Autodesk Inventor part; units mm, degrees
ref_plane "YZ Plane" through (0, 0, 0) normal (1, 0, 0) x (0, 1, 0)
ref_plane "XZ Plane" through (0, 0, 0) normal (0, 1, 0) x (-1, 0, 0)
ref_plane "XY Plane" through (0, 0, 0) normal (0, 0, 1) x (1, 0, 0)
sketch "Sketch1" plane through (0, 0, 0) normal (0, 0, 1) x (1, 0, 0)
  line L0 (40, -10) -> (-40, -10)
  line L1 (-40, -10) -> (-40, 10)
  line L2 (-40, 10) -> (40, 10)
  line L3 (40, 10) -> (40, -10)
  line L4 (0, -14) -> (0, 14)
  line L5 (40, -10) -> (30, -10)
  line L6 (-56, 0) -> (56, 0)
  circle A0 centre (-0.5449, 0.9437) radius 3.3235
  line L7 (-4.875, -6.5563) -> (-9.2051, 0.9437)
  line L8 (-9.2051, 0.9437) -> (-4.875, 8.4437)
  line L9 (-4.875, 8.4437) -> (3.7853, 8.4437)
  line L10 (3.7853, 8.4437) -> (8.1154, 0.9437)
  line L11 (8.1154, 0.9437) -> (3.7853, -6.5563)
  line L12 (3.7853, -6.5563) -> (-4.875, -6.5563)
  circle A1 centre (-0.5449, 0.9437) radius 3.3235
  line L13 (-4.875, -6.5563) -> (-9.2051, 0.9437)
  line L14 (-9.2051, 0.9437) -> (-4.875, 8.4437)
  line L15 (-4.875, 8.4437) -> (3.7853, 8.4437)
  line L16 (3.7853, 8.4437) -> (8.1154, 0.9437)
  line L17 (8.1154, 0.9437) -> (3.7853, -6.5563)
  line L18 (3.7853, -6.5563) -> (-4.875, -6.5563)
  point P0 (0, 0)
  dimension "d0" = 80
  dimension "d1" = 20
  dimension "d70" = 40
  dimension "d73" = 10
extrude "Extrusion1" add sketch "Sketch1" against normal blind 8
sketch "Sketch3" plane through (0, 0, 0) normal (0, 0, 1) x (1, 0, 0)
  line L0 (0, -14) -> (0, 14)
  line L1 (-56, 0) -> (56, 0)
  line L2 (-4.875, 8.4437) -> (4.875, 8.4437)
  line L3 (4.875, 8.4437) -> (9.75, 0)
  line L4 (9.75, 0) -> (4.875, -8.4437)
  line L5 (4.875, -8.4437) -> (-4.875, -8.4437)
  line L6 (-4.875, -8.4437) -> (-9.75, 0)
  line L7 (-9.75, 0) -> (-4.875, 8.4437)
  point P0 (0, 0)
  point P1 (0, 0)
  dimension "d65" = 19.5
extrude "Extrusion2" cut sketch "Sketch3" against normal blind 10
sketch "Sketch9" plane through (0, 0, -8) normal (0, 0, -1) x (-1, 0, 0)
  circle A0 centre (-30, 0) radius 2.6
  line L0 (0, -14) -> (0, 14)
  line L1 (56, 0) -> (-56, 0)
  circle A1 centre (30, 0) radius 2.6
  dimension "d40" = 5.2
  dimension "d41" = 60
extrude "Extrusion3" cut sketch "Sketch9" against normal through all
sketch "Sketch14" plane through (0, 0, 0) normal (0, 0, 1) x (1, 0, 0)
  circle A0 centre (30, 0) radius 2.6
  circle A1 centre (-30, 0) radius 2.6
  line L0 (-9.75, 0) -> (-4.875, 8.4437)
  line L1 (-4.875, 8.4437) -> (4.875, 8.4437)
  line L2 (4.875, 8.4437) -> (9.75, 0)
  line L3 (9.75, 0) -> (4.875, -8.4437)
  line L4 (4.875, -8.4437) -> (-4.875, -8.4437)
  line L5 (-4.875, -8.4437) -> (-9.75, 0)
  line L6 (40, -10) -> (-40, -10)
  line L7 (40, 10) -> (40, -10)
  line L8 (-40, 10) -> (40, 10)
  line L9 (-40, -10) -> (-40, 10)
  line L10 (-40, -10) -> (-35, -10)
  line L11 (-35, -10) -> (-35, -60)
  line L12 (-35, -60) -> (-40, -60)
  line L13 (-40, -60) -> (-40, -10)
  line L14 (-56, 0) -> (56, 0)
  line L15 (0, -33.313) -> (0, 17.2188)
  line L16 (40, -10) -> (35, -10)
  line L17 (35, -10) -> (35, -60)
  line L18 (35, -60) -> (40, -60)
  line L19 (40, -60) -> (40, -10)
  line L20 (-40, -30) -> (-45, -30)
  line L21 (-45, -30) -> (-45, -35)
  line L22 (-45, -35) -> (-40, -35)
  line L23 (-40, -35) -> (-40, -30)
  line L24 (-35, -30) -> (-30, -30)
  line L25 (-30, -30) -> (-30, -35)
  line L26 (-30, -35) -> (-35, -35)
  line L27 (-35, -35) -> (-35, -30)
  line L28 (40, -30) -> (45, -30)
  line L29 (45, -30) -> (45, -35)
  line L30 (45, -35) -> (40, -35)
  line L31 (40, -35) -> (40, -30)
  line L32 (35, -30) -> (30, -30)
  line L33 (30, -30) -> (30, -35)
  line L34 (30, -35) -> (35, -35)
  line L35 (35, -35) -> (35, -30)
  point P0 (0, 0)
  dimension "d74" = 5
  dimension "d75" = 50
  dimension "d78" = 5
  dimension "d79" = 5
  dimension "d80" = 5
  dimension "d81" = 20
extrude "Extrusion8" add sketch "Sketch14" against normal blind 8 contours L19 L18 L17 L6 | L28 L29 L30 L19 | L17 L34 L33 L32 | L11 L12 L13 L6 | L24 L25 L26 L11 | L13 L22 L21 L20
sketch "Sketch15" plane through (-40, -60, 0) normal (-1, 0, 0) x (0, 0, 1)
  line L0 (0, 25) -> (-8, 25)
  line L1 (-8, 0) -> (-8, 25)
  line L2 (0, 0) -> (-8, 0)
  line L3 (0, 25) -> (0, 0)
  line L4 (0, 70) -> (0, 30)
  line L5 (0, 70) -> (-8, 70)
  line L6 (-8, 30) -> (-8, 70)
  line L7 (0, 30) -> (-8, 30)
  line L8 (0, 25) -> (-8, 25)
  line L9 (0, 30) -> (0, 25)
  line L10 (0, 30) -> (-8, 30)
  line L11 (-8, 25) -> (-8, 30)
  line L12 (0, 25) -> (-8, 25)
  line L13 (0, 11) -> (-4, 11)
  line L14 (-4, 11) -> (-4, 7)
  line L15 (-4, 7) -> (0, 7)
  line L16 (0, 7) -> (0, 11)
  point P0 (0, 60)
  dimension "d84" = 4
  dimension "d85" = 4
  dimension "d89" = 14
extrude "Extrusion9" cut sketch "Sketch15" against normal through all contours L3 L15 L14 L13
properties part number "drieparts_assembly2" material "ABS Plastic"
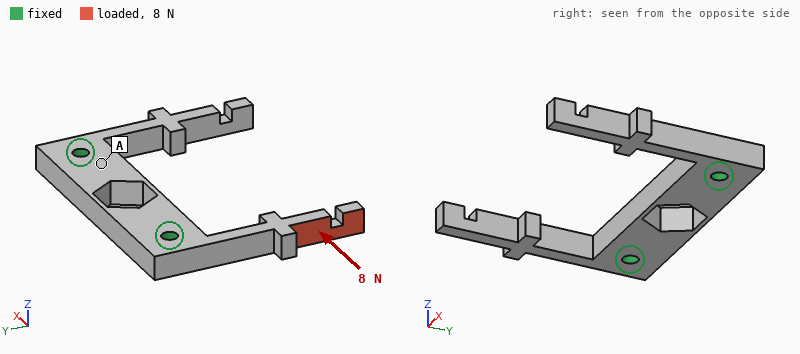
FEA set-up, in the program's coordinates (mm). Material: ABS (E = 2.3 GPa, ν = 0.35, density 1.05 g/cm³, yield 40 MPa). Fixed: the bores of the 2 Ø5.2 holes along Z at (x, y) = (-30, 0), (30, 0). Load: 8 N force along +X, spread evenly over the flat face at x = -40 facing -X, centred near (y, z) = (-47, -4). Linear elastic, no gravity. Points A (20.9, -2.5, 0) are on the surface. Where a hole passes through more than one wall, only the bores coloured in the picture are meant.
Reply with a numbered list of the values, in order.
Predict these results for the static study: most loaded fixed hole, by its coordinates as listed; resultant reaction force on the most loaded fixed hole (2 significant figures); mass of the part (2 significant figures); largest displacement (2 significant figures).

1. (-30, 0)
2. 7.3 N
3. 16 g
4. 1.3 mm
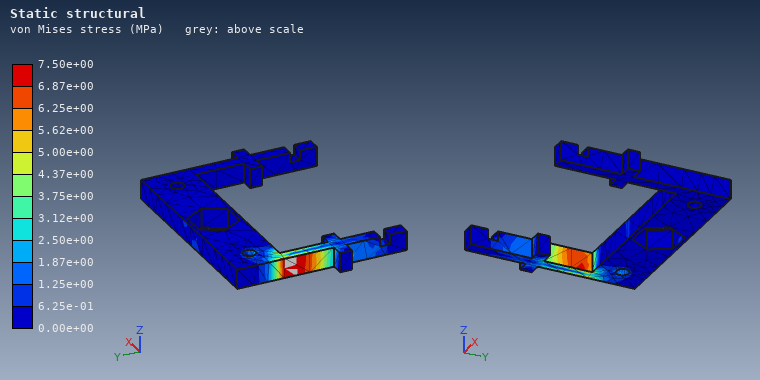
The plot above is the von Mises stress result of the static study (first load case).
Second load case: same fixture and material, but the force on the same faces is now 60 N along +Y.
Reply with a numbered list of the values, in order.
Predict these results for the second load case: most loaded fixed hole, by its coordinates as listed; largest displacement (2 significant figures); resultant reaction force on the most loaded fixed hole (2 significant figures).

1. (-30, 0)
2. 1.1 mm
3. 62 N
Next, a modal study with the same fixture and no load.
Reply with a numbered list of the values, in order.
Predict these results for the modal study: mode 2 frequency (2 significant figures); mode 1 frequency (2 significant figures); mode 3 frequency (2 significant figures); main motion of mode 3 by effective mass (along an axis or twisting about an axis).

1. 430 Hz
2. 430 Hz
3. 590 Hz
4. along Z
